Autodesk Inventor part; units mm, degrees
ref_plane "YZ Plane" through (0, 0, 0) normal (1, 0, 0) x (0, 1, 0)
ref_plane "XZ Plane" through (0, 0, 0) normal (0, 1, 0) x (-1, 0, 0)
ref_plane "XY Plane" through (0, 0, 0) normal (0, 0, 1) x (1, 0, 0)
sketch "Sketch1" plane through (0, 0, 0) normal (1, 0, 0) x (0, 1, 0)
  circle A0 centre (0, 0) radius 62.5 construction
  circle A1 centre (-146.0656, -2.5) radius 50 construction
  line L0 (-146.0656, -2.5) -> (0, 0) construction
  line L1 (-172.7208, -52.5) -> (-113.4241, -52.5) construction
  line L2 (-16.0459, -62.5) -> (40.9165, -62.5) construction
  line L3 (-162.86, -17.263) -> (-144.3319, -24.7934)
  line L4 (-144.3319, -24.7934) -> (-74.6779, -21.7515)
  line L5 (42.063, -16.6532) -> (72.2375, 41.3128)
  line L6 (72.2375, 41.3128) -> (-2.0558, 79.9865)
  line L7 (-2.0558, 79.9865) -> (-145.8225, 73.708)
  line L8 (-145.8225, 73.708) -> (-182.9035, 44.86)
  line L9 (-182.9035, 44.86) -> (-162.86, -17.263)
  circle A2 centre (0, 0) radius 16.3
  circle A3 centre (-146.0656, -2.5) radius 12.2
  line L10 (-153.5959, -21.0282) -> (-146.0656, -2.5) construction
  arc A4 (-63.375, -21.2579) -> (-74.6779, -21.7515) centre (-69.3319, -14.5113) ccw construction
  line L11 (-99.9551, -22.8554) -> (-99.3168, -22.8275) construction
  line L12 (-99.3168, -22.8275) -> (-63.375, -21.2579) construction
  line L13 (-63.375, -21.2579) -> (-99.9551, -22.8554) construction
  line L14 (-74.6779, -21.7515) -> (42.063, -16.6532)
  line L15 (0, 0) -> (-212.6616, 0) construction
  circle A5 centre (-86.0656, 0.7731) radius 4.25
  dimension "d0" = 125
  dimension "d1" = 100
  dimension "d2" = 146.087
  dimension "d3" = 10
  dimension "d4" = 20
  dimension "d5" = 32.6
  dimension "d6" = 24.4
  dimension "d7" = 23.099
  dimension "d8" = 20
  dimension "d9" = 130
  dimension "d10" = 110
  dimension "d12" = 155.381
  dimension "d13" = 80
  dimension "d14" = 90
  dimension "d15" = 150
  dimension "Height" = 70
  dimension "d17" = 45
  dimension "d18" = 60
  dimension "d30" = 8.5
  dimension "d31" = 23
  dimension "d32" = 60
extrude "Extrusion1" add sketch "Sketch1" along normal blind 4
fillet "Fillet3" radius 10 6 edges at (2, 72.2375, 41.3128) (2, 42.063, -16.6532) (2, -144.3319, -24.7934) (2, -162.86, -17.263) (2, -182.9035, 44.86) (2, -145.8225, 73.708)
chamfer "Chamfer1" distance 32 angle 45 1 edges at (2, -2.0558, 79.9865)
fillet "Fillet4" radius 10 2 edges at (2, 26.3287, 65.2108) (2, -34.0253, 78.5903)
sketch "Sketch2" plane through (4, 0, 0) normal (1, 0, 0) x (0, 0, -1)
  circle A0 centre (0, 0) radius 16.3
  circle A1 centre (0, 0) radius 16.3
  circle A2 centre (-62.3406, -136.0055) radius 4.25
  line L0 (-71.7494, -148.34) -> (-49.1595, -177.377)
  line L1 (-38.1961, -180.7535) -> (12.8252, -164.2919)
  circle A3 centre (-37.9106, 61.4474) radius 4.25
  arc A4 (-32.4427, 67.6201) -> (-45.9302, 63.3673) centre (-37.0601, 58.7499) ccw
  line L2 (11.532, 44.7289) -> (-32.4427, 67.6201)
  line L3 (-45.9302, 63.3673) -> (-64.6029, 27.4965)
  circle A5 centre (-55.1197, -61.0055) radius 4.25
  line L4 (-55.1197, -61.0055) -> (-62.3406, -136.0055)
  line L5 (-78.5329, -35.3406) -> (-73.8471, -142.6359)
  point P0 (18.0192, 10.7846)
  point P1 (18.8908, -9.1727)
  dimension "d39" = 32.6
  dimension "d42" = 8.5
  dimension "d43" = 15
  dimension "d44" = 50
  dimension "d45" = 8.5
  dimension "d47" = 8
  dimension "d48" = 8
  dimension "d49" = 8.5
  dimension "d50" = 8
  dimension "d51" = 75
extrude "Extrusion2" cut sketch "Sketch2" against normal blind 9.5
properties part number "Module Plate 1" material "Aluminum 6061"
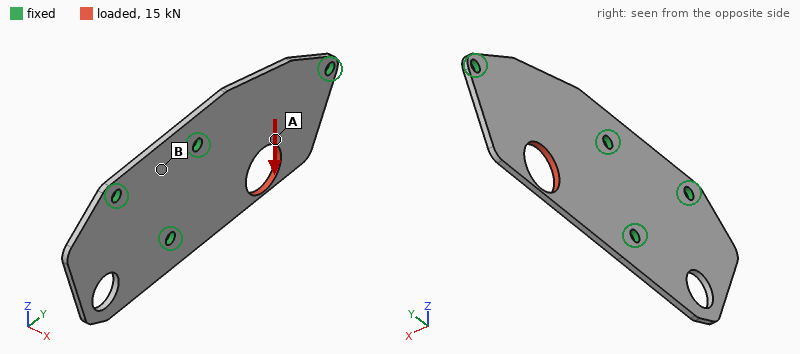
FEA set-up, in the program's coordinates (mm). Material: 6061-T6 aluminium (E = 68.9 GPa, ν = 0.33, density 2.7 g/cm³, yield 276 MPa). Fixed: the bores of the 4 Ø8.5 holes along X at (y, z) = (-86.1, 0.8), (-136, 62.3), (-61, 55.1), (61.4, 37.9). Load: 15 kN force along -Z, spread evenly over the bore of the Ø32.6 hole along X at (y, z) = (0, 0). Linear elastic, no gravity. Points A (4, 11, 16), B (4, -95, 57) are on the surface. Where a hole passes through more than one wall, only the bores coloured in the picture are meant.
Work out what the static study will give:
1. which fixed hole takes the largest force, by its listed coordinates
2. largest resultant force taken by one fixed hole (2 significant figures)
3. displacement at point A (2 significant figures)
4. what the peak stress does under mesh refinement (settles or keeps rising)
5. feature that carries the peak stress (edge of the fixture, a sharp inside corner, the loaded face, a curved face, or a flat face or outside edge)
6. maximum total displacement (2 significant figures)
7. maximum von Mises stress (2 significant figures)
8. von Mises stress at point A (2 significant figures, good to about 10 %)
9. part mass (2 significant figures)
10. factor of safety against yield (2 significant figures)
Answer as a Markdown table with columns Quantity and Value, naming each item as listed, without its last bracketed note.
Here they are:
| Quantity | Value |
|---|---|
| which fixed hole takes the largest force, by its listed coordinates | (-61, 55.1) |
| largest resultant force taken by one fixed hole | 8.4 kN |
| displacement at point A | 0.089 mm |
| what the peak stress does under mesh refinement | settles |
| feature that carries the peak stress | a flat face or outside edge |
| maximum total displacement | 0.23 mm |
| maximum von Mises stress | 580 MPa |
| von Mises stress at point A | 51 MPa |
| part mass | 210 g |
| factor of safety against yield | 0.48 |
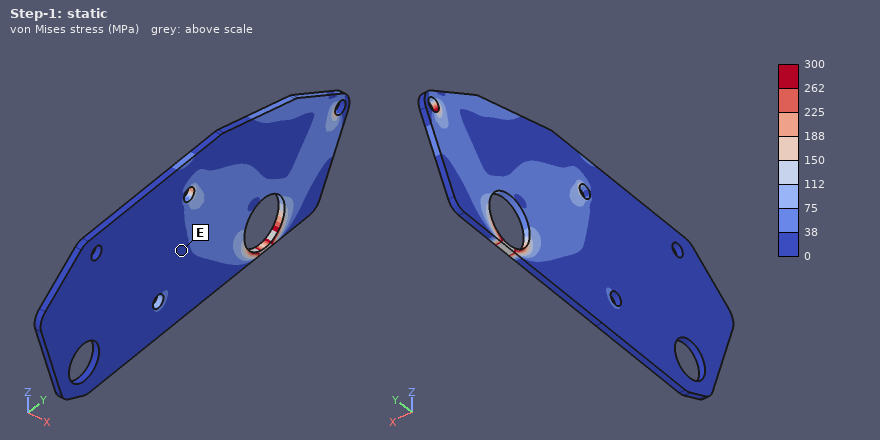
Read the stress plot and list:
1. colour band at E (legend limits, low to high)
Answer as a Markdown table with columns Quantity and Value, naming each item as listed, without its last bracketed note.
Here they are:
| Quantity | Value |
|---|---|
| colour band at E | 0 to 38 MPa |
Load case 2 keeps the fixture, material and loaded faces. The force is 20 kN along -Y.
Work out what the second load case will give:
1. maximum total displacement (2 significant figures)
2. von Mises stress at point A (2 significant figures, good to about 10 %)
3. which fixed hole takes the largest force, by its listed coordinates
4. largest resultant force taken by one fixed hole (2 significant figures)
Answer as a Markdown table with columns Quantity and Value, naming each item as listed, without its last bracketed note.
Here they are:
| Quantity | Value |
|---|---|
| maximum total displacement | 0.15 mm |
| von Mises stress at point A | 100 MPa |
| which fixed hole takes the largest force, by its listed coordinates | (61.4, 37.9) |
| largest resultant force taken by one fixed hole | 8.3 kN |
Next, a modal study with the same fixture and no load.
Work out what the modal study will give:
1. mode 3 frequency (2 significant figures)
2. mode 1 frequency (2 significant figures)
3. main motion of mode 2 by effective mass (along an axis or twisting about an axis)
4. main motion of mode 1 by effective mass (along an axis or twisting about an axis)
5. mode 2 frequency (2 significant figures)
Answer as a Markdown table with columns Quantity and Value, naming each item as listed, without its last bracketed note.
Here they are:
| Quantity | Value |
|---|---|
| mode 3 frequency | 1400 Hz |
| mode 1 frequency | 910 Hz |
| main motion of mode 2 by effective mass | along X |
| main motion of mode 1 by effective mass | along X |
| mode 2 frequency | 970 Hz |
